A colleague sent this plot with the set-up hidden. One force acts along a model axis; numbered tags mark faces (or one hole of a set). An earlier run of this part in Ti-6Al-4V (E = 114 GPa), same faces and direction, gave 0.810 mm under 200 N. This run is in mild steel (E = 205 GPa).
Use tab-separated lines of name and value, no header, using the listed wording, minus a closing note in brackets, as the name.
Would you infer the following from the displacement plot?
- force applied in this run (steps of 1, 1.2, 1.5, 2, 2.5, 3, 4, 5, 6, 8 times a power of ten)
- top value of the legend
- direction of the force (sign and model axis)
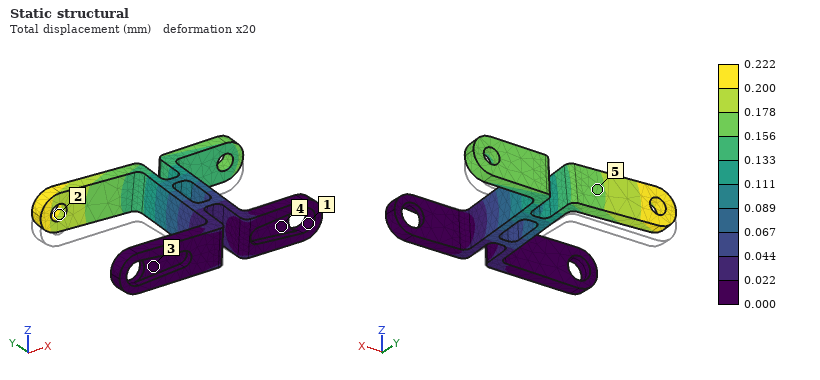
force applied in this run	100 N
top value of the legend	0.222 mm
direction of the force	+Z
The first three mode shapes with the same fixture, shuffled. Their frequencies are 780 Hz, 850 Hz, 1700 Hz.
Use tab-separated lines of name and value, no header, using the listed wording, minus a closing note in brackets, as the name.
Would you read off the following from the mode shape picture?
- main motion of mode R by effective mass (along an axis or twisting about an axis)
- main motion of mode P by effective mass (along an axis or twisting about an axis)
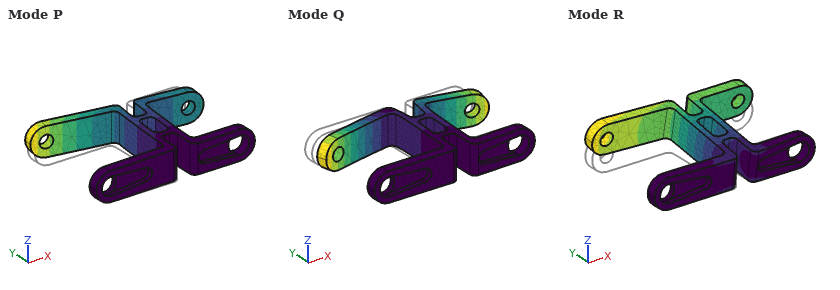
main motion of mode R by effective mass	along Z
main motion of mode P by effective mass	along X
